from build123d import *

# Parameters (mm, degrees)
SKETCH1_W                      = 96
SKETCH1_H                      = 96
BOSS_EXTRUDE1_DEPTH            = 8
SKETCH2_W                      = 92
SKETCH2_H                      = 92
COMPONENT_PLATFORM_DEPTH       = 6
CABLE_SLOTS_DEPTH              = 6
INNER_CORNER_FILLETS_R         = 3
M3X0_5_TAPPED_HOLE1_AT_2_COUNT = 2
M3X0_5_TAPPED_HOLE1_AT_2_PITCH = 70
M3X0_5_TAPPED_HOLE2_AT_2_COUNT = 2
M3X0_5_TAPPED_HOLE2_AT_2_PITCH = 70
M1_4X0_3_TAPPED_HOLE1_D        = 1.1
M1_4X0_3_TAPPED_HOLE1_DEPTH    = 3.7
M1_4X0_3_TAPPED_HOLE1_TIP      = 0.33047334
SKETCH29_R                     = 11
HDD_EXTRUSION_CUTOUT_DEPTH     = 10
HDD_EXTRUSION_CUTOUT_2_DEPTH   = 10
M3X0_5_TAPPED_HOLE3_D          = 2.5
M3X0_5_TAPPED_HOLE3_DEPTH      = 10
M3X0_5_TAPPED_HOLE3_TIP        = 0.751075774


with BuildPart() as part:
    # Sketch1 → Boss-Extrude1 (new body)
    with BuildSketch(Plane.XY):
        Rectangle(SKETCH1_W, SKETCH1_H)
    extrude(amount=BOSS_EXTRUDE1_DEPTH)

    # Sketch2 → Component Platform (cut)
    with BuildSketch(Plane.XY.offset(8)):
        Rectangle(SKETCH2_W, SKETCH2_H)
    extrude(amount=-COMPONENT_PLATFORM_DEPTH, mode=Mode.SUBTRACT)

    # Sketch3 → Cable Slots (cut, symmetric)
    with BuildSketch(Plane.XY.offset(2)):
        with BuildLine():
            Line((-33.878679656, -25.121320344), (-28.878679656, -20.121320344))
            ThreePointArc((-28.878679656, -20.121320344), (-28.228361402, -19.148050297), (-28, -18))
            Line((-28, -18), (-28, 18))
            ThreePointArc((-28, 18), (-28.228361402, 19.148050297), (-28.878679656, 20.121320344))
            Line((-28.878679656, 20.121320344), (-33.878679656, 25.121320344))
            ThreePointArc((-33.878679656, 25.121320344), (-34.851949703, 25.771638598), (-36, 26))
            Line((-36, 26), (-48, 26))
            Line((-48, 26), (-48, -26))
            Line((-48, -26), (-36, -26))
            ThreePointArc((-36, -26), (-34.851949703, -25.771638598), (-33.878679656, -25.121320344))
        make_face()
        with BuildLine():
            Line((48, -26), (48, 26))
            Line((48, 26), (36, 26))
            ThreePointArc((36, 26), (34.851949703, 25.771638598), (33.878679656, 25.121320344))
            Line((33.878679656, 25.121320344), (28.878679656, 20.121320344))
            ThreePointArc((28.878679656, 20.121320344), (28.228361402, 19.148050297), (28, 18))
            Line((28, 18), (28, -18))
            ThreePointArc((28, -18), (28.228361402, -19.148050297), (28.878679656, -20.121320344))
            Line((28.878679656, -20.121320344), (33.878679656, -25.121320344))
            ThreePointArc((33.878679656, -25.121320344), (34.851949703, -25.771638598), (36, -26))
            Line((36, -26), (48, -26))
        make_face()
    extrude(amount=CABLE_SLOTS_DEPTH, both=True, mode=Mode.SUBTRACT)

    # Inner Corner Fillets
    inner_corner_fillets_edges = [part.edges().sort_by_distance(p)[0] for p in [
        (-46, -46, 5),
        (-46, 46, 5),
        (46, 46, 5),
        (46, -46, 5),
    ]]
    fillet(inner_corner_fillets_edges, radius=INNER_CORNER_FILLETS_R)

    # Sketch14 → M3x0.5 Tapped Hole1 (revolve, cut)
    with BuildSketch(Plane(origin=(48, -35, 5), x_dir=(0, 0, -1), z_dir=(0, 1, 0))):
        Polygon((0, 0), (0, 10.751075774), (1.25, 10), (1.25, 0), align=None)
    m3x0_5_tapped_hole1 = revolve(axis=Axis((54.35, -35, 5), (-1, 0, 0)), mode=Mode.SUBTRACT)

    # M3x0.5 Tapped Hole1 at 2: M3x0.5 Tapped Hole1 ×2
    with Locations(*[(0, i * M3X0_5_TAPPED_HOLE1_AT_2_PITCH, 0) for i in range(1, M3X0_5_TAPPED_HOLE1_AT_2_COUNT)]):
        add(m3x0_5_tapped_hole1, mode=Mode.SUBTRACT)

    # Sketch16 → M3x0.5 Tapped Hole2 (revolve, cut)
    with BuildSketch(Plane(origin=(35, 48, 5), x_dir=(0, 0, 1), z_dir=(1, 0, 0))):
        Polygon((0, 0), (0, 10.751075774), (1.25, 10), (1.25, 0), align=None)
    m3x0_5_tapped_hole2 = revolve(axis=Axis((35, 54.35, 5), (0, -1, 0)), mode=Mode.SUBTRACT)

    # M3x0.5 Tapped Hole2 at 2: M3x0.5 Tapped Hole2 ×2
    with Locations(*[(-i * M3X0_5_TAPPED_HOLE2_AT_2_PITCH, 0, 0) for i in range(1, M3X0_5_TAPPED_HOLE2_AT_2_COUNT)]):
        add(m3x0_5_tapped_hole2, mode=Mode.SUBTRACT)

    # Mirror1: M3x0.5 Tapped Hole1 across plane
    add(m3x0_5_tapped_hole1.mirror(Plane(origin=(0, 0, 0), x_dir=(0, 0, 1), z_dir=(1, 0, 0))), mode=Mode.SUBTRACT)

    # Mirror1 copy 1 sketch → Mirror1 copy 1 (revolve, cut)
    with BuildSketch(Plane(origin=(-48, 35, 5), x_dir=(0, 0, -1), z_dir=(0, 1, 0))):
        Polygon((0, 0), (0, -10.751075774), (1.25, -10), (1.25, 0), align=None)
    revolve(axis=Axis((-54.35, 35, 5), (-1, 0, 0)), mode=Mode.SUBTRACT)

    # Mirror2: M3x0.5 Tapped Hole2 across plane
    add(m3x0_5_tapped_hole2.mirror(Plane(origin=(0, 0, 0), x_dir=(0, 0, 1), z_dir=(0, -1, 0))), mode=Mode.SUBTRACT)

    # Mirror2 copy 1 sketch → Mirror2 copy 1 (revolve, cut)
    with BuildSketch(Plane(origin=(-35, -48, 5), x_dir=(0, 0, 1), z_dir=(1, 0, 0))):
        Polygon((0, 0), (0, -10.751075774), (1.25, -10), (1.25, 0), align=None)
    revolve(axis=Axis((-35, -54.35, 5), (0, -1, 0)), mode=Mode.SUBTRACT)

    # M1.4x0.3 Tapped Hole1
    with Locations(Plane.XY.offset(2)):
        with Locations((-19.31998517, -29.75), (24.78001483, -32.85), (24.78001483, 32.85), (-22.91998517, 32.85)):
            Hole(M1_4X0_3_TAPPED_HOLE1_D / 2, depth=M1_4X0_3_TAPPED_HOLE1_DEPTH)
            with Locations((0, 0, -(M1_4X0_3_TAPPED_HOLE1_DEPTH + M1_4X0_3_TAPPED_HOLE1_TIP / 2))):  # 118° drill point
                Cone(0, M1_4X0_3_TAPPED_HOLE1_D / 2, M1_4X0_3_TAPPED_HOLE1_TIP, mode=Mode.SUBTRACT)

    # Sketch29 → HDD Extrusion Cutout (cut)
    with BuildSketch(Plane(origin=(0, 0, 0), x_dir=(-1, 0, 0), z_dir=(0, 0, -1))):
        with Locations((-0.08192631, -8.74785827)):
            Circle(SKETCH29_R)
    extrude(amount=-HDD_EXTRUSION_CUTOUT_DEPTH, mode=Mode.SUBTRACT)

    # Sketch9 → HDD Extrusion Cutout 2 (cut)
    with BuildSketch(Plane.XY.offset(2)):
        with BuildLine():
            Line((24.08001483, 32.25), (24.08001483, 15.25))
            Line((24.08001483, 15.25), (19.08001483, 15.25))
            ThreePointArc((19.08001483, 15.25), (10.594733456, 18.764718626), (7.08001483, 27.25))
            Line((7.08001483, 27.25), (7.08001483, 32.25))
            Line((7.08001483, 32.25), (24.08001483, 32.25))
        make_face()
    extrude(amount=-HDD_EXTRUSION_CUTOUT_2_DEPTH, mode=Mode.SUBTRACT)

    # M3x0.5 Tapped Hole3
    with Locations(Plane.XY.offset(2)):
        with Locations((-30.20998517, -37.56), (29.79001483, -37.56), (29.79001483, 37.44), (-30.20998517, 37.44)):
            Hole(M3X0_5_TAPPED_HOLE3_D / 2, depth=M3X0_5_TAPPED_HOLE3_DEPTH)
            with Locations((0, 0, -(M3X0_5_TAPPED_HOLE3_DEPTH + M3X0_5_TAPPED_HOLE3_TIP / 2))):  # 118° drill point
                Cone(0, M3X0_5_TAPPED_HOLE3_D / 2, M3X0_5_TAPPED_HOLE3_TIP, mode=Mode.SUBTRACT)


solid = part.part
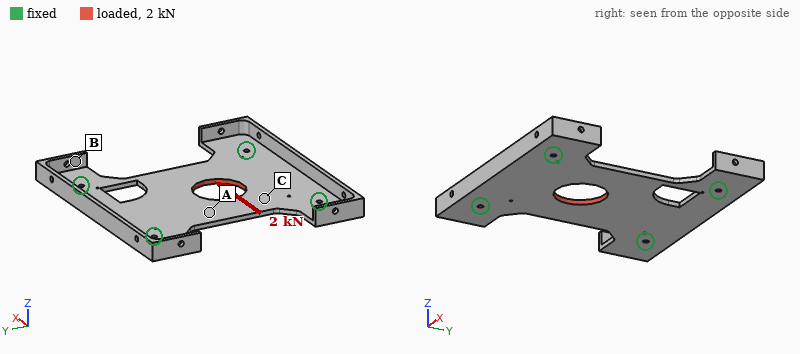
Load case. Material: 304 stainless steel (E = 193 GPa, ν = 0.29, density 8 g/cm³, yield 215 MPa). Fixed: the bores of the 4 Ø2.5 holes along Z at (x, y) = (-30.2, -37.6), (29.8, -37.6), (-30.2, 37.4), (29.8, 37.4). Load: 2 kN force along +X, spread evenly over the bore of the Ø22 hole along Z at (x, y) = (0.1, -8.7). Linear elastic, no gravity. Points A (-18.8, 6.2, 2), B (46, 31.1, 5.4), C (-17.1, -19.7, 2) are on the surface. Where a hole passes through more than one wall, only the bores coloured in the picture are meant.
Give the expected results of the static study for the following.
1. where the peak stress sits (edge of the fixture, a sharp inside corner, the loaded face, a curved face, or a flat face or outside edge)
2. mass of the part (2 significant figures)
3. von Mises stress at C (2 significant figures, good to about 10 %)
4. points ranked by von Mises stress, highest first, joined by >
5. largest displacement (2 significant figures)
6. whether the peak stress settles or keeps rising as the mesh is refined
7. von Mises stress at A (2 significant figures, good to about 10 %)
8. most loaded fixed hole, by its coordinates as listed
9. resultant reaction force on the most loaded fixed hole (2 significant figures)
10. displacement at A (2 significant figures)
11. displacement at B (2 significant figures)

edge of the fixture
130 g
20 MPa
C > A > B
6.9 µm
keeps rising
12 MPa
(-30.2, -37.6)
800 N
5.7 µm
1.1 µm
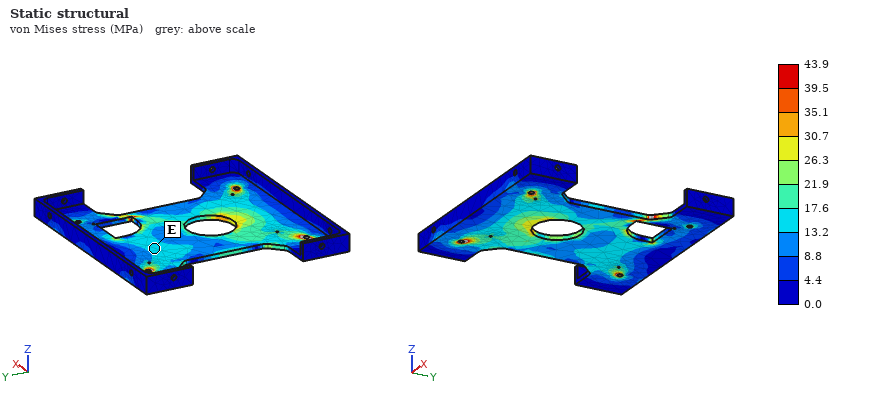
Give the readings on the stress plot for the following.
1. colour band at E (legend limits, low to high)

13.2 to 17.6 MPa
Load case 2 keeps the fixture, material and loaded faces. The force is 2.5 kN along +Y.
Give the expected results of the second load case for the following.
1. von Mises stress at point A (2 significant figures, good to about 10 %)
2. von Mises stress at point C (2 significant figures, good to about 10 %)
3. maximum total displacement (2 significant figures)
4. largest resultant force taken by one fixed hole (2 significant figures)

15 MPa
17 MPa
8.3 µm
840 N
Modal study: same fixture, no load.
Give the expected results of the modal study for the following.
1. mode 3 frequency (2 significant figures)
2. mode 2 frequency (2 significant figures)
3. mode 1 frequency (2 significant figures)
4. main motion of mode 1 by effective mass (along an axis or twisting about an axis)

3200 Hz
2500 Hz
1400 Hz
along Z
